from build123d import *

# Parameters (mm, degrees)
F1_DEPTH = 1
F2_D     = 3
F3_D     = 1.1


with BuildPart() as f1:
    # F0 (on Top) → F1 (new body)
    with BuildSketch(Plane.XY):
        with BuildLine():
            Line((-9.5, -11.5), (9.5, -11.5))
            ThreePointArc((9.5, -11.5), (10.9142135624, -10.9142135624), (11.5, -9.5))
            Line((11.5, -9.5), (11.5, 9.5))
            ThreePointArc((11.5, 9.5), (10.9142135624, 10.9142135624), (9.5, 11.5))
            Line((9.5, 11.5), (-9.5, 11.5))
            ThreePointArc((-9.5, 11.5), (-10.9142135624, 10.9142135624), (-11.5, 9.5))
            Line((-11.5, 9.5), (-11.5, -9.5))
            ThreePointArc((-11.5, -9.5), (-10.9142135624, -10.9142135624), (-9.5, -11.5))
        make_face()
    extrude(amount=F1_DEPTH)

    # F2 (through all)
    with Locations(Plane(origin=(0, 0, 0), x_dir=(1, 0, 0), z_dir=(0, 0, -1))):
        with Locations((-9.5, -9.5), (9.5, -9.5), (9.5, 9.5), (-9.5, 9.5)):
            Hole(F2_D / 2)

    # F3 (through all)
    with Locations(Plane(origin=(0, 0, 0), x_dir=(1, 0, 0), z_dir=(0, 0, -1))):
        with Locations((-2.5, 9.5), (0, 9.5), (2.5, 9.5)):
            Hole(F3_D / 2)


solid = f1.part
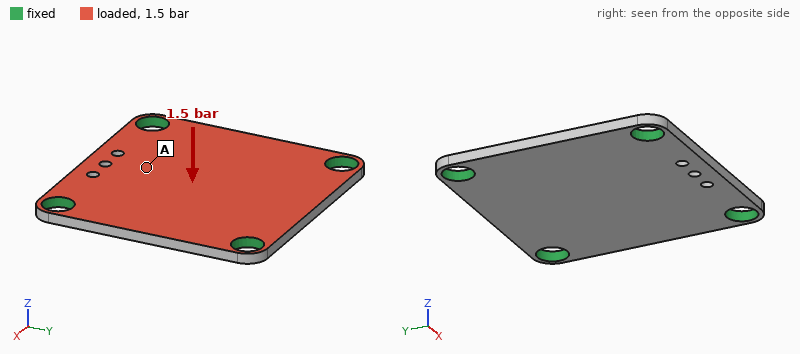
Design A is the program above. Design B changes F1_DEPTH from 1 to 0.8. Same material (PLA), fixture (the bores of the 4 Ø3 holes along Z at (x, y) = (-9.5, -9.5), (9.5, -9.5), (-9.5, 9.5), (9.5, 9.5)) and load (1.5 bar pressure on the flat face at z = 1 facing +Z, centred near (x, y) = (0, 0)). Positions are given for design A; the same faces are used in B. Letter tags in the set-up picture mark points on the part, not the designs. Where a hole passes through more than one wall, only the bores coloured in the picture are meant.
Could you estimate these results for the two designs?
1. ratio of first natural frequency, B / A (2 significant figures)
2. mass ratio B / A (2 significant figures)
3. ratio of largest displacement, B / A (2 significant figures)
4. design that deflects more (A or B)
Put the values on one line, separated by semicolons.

0.81; 0.80; 1.9; B
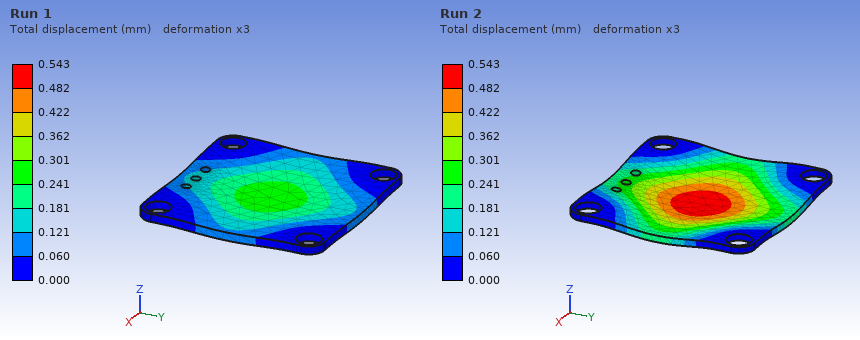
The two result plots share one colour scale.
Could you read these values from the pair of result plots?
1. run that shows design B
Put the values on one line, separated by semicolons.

Run 2
